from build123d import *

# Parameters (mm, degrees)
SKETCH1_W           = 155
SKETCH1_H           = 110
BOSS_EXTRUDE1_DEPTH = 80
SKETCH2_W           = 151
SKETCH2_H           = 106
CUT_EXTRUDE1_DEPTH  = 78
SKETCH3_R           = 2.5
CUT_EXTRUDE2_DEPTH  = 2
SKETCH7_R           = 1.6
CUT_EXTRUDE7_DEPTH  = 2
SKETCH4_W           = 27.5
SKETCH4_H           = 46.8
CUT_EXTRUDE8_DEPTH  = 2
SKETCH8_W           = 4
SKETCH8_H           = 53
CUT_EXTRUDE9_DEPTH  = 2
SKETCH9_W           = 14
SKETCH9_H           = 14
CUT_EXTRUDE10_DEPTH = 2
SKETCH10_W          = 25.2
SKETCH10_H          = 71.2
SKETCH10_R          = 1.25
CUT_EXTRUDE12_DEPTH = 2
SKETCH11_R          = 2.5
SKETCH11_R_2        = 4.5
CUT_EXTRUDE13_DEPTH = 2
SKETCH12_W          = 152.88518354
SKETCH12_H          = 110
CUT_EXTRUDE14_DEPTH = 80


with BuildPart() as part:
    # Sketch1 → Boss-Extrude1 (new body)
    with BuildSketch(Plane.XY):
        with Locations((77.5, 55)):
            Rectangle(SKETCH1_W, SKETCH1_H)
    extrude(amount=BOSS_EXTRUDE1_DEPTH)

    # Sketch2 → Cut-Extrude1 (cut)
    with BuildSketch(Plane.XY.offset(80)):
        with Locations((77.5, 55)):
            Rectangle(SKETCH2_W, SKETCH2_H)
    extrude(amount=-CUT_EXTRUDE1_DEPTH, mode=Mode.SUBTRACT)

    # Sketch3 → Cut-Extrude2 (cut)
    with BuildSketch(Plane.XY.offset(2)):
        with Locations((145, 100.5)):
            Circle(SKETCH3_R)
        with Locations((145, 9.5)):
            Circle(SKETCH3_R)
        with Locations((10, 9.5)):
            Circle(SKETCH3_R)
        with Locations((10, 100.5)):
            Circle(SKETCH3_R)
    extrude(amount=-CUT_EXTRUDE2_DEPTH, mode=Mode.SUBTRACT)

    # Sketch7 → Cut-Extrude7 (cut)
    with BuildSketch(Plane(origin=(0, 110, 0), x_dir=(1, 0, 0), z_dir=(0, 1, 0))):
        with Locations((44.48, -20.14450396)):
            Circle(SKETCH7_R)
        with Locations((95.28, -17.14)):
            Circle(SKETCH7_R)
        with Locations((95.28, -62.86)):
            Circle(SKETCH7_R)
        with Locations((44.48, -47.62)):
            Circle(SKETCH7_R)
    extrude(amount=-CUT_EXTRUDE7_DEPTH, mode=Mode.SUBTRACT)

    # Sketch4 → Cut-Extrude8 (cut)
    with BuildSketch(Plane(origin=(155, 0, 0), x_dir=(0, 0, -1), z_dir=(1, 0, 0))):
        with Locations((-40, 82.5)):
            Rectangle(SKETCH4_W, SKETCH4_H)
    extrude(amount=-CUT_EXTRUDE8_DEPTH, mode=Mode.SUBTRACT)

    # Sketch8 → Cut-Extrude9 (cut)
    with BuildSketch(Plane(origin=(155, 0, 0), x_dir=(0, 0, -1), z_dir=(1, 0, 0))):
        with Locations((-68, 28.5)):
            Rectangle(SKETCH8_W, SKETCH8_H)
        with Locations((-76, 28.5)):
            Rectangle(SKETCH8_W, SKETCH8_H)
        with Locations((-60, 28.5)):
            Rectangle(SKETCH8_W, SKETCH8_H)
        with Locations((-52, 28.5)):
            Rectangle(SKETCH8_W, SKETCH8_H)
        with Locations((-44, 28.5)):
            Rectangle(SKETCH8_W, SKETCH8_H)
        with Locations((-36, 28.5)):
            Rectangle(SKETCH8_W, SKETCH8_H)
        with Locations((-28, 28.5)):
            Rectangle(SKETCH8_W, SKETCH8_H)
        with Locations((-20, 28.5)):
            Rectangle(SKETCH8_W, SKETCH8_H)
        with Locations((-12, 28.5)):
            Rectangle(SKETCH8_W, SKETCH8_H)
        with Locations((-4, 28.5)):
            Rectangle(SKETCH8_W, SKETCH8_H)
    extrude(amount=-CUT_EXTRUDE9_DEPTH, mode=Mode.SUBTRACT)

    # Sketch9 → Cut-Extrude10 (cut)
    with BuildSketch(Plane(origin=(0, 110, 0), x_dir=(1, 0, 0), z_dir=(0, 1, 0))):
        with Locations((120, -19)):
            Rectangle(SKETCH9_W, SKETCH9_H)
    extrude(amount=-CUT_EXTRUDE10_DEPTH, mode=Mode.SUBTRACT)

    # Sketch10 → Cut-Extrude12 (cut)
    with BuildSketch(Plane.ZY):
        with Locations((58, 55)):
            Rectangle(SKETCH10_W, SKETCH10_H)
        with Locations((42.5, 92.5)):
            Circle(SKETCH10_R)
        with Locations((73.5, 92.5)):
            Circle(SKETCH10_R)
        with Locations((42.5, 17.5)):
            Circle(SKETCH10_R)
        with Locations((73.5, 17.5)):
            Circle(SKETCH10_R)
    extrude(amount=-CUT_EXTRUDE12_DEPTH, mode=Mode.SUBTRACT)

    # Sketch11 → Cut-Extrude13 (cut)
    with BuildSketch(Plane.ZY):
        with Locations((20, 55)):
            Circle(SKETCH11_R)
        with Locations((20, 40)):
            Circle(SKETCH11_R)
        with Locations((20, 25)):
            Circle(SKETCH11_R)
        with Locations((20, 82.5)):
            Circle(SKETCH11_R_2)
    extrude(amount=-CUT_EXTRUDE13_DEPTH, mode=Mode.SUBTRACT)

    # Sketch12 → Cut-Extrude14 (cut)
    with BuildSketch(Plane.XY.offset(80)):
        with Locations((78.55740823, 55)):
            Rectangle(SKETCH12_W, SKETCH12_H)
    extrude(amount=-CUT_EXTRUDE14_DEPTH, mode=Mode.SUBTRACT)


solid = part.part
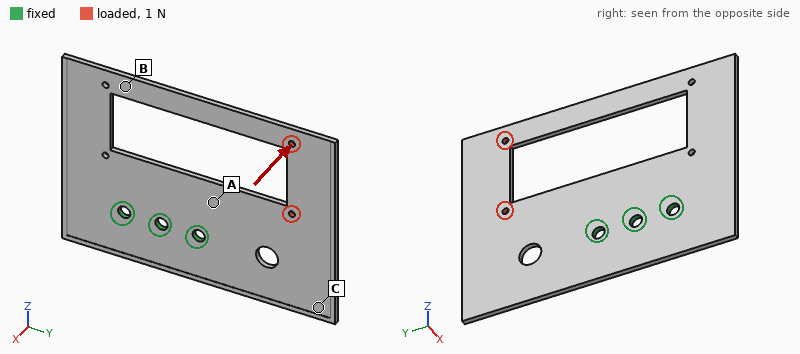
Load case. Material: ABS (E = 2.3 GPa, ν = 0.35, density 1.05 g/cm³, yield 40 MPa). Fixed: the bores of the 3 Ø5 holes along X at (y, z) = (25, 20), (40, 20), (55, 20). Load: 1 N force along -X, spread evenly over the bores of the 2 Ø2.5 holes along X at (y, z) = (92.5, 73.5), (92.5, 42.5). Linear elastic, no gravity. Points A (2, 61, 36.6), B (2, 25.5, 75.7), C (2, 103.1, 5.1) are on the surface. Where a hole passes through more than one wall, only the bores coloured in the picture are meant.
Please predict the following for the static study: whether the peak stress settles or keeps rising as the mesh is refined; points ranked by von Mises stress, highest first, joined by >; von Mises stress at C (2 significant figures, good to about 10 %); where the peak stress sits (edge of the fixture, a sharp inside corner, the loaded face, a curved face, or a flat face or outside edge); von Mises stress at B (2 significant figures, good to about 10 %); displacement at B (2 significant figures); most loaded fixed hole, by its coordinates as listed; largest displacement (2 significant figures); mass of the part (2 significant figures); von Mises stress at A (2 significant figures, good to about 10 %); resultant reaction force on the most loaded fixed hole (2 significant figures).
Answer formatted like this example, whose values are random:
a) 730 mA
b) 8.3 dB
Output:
a) keeps rising
b) A > B > C
c) 0.26 MPa
d) edge of the fixture
e) 0.72 MPa
f) 0.26 mm
g) (55, 20)
h) 1.4 mm
i) 14 g
j) 1.1 MPa
k) 1.8 N
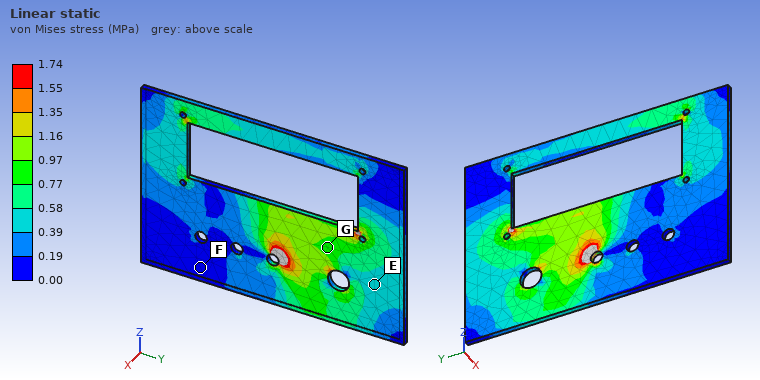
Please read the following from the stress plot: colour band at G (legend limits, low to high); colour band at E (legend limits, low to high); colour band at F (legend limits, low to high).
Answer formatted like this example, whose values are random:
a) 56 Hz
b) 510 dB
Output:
a) 0.77 to 0.97 MPa
b) 0.39 to 0.58 MPa
c) 0.00 to 0.19 MPa
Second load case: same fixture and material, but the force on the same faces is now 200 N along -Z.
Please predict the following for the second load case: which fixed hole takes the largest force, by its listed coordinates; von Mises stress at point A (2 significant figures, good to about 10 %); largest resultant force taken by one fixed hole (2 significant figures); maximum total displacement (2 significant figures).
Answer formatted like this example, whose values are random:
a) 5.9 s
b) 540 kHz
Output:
a) (55, 20)
b) 5.6 MPa
c) 420 N
d) 0.67 mm
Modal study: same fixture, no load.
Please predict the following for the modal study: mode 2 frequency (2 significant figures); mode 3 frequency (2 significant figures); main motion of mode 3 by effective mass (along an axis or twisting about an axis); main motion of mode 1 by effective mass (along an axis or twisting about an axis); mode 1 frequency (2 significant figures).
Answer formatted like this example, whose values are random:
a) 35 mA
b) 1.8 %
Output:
a) 130 Hz
b) 200 Hz
c) along X
d) along X
e) 91 Hz
